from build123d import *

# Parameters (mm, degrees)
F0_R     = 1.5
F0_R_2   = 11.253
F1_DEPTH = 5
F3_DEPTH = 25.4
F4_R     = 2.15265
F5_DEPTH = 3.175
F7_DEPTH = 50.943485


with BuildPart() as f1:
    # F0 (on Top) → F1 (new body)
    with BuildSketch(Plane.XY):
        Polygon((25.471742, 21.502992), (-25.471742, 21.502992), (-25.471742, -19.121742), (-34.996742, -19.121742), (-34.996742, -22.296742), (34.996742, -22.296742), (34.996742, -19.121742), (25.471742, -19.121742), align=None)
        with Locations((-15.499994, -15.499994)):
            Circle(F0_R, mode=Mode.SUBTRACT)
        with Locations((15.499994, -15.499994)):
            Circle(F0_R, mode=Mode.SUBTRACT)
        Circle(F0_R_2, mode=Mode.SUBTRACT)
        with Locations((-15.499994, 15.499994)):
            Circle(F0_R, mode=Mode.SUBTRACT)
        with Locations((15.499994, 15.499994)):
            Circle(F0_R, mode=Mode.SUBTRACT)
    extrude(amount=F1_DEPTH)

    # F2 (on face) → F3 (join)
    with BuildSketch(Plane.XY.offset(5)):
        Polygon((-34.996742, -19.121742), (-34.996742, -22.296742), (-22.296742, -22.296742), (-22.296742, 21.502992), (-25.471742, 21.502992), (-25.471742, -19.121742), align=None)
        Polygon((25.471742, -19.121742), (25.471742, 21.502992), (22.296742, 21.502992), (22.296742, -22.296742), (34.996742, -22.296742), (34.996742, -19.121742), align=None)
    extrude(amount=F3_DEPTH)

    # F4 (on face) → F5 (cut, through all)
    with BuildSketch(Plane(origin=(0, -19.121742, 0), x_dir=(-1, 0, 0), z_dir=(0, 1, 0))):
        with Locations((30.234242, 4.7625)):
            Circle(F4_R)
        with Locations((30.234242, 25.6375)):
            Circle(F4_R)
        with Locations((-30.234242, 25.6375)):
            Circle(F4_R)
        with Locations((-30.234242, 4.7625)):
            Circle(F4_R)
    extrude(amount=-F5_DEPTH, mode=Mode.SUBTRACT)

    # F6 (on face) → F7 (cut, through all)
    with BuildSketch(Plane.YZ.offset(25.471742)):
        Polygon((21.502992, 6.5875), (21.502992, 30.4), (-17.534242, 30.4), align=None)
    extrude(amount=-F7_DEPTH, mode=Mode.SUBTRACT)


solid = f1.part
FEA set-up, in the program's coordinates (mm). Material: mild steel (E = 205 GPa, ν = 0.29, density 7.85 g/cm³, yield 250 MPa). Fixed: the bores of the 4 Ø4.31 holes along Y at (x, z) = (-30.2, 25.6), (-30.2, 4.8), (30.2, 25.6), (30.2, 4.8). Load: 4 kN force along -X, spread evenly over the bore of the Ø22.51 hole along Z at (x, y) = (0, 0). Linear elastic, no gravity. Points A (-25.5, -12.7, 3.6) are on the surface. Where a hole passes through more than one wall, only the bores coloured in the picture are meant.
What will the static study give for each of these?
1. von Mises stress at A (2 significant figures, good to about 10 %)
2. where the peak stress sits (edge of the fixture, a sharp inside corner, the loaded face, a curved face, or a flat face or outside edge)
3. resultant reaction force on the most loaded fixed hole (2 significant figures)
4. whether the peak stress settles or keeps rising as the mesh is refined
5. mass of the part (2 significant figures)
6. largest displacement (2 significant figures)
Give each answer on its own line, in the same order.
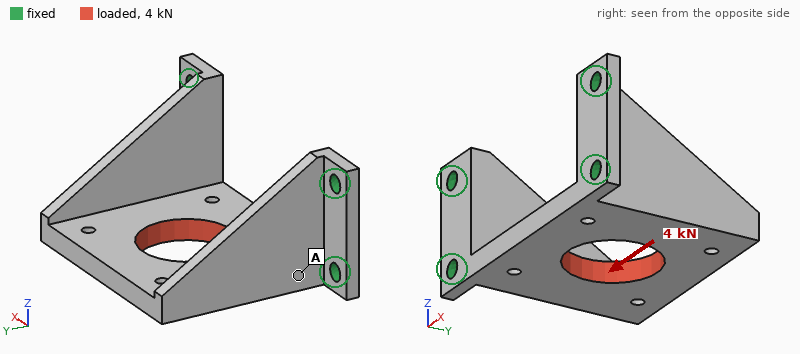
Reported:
34 MPa
edge of the fixture
2.5 kN
keeps rising
120 g
32 µm
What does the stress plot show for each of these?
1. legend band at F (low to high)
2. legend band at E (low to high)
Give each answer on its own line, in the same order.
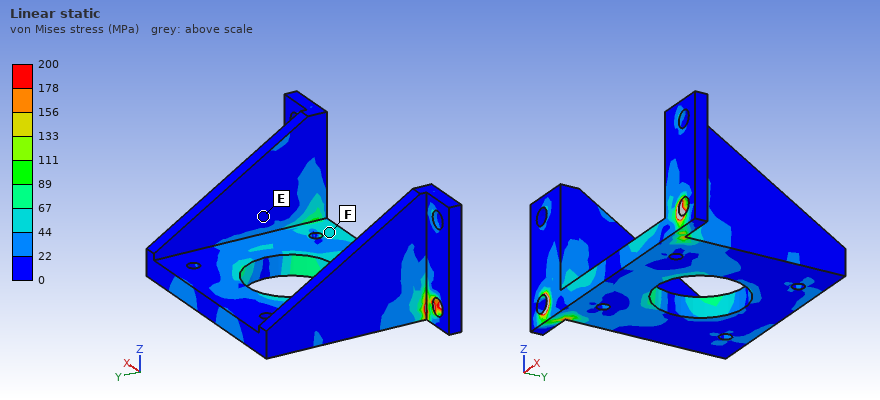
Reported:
44 to 67 MPa
0 to 22 MPa
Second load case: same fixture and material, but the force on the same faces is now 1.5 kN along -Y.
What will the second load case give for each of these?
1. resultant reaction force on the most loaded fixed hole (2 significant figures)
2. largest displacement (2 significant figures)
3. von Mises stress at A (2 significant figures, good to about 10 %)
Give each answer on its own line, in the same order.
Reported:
900 N
14 µm
20 MPa
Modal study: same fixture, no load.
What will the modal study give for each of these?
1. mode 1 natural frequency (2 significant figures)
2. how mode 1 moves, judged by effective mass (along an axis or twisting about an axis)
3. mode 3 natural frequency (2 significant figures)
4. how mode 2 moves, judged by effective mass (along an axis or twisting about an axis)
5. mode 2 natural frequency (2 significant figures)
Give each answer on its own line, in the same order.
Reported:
4100 Hz
along Z
8100 Hz
along X
5900 Hz
